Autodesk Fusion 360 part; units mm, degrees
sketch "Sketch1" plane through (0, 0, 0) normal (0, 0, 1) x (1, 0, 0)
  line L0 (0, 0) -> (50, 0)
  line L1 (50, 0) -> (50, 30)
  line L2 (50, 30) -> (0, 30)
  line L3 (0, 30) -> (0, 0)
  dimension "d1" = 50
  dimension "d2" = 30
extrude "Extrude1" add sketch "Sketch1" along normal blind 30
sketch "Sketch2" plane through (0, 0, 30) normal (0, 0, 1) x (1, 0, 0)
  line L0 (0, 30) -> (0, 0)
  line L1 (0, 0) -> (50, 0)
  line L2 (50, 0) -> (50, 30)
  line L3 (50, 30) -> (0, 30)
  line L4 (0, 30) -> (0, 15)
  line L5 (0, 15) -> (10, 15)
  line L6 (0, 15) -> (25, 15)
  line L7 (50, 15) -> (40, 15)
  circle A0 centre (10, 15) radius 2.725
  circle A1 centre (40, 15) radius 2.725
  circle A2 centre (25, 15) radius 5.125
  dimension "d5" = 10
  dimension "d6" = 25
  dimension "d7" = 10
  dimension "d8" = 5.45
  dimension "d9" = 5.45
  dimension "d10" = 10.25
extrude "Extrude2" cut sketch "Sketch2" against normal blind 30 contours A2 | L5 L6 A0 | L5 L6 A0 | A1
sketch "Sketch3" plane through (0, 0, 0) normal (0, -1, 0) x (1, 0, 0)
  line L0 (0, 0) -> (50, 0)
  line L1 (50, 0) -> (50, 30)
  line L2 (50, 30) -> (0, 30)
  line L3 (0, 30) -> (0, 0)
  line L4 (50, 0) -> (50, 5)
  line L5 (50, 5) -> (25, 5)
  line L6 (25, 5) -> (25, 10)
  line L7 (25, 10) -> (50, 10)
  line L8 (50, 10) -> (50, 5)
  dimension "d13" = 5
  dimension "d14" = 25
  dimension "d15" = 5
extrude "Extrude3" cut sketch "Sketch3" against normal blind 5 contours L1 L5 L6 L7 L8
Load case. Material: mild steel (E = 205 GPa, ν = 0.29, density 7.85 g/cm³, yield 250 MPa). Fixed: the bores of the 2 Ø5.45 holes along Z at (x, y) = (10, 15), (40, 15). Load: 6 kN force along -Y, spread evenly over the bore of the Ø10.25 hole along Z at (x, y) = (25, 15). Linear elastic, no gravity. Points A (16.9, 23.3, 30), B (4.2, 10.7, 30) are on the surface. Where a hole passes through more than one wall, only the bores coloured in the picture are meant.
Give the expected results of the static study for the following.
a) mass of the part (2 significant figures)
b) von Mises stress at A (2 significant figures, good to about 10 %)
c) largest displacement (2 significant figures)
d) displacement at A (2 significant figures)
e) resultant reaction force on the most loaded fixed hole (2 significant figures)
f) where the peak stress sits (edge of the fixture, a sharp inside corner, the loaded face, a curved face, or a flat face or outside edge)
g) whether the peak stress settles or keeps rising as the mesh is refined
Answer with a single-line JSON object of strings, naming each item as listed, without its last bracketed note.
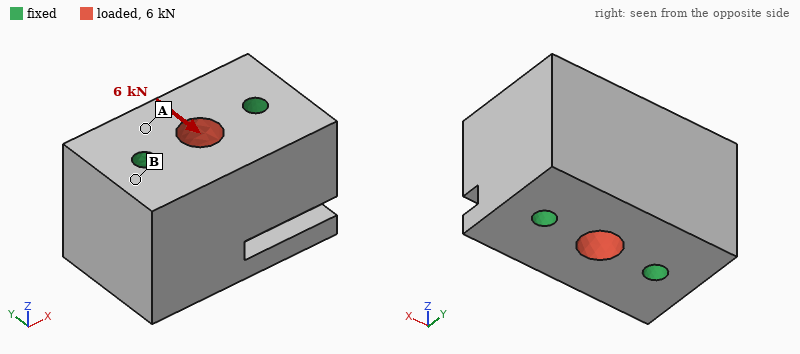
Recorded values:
{"mass of the part": "320 g", "von Mises stress at A": "6.7 MPa", "largest displacement": "0.88 µm", "displacement at A": "0.46 µm", "resultant reaction force on the most loaded fixed hole": "3.0 kN", "where the peak stress sits": "edge of the fixture", "whether the peak stress settles or keeps rising as the mesh is refined": "keeps rising"}
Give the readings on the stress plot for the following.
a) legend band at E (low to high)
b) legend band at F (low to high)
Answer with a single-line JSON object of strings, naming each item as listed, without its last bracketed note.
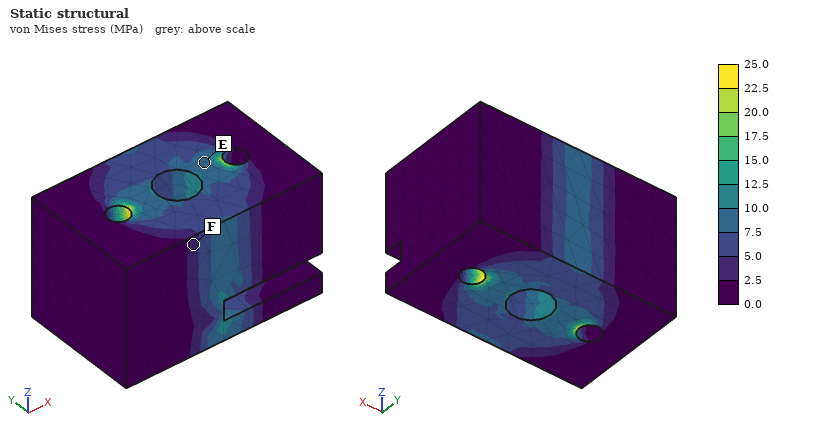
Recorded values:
{"legend band at E": "7.5 to 10.0 MPa", "legend band at F": "2.5 to 5.0 MPa"}
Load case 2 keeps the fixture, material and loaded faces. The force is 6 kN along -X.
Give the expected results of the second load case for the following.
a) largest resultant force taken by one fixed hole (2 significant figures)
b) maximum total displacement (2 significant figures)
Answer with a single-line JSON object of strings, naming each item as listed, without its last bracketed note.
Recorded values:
{"largest resultant force taken by one fixed hole": "3.0 kN", "maximum total displacement": "0.45 µm"}
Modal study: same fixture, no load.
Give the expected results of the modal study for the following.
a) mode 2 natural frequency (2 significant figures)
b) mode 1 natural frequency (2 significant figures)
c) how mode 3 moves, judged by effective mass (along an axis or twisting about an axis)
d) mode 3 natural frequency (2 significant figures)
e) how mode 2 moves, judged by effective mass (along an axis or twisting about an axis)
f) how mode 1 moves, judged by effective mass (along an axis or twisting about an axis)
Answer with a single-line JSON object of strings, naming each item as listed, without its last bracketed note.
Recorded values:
{"mode 2 natural frequency": "36 kHz", "mode 1 natural frequency": "34 kHz", "how mode 3 moves, judged by effective mass": "along Z", "mode 3 natural frequency": "38 kHz", "how mode 2 moves, judged by effective mass": "twisting about X", "how mode 1 moves, judged by effective mass": "twisting about Z"}
